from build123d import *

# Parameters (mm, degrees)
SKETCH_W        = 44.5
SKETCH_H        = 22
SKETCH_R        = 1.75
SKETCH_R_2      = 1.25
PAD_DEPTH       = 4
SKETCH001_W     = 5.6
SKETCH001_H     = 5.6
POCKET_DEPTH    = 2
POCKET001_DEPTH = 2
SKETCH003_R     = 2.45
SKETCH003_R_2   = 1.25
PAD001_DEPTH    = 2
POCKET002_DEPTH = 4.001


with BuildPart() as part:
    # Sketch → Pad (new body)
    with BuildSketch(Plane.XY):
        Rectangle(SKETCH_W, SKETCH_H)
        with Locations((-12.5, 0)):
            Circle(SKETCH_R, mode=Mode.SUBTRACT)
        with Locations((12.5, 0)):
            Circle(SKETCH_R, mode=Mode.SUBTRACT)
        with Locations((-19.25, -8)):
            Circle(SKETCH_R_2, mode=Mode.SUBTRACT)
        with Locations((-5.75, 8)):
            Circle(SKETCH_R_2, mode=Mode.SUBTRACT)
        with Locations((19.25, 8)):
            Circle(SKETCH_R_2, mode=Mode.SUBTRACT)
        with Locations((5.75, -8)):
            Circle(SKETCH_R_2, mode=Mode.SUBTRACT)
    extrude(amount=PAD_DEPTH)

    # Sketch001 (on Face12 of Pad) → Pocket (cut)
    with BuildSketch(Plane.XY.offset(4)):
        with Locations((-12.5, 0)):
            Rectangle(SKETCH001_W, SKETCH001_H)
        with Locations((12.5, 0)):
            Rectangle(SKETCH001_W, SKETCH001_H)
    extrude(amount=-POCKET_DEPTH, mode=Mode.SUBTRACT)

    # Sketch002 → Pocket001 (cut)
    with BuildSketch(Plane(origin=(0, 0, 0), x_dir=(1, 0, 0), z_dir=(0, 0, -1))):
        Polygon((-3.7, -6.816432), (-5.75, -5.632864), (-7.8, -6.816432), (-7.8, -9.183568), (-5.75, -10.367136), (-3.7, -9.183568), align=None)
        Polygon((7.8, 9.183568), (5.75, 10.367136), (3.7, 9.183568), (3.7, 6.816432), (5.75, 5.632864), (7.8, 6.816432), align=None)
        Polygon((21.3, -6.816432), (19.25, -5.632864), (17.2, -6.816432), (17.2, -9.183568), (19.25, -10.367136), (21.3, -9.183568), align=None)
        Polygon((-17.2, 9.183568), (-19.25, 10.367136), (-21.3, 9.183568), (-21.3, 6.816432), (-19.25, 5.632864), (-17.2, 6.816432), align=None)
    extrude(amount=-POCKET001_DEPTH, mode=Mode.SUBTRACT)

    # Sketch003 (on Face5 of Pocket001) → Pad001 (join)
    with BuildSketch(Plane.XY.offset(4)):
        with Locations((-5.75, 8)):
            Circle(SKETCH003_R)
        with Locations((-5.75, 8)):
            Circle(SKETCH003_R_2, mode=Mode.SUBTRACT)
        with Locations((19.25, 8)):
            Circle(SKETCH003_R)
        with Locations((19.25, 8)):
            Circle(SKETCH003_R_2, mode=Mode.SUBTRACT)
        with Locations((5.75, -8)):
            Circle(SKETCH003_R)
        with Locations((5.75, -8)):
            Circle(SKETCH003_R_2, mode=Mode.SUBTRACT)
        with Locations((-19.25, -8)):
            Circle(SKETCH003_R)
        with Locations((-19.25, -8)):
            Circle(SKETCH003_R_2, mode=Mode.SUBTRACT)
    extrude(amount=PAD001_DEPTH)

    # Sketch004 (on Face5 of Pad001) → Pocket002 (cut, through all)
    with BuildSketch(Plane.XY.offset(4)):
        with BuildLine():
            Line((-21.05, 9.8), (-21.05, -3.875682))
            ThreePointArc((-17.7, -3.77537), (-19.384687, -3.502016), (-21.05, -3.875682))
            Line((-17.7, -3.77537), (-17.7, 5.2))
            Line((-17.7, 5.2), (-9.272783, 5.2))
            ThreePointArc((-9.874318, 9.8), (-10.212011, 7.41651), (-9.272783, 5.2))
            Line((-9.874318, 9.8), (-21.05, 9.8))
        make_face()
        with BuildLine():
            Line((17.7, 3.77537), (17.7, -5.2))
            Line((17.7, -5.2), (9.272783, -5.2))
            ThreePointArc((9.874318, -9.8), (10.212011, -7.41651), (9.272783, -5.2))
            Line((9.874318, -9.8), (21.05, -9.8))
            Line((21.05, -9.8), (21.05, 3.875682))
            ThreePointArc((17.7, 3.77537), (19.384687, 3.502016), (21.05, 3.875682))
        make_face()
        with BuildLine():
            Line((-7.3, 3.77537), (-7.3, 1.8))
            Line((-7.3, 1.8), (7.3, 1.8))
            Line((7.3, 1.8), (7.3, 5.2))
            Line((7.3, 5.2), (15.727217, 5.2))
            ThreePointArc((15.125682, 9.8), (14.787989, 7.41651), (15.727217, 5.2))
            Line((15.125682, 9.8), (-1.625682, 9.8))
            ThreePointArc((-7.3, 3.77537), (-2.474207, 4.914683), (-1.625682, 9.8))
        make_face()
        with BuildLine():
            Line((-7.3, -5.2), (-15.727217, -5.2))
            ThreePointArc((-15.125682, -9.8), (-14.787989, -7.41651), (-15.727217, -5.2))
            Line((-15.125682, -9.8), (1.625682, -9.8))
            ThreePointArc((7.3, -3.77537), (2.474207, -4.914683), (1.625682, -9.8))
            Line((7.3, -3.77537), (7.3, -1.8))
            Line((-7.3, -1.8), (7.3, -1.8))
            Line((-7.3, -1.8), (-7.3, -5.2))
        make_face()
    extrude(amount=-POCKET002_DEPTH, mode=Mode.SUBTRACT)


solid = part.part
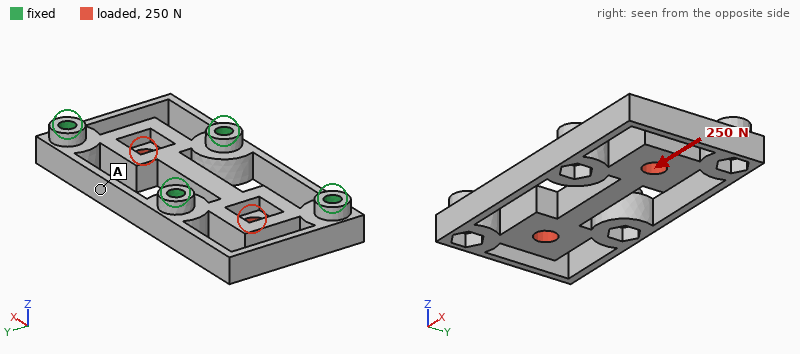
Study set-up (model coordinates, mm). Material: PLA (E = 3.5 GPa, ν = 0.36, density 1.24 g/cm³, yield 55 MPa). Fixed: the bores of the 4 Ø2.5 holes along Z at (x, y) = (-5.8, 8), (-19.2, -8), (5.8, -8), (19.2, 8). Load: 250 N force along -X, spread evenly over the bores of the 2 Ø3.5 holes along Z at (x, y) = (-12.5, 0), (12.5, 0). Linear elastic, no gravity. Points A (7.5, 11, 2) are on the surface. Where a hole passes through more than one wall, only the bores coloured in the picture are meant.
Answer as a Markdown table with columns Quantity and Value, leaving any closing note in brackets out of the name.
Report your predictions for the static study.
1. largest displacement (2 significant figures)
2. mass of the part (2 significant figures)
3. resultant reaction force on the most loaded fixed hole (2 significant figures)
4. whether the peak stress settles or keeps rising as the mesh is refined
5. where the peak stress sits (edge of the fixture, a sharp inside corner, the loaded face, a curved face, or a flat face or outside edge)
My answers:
| Quantity | Value |
|---|---|
| largest displacement | 56 µm |
| mass of the part | 2.6 g |
| resultant reaction force on the most loaded fixed hole | 64 N |
| whether the peak stress settles or keeps rising as the mesh is refined | keeps rising |
| where the peak stress sits | edge of the fixture |
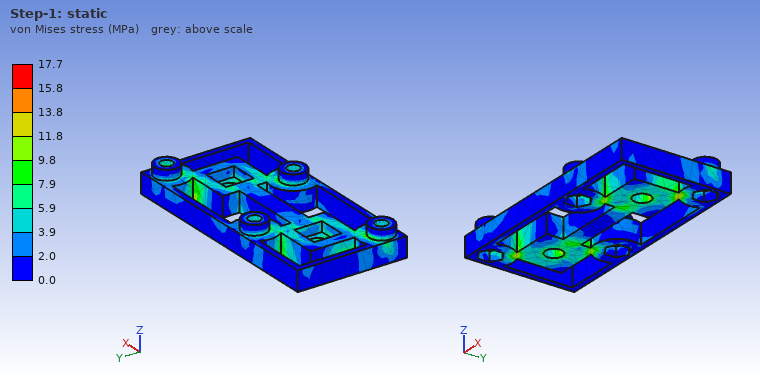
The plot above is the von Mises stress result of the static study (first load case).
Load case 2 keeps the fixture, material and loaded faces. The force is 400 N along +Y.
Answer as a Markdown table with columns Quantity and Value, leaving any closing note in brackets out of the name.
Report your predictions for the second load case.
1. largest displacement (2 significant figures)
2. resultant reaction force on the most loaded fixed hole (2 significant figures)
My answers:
| Quantity | Value |
|---|---|
| largest displacement | 82 µm |
| resultant reaction force on the most loaded fixed hole | 100 N |
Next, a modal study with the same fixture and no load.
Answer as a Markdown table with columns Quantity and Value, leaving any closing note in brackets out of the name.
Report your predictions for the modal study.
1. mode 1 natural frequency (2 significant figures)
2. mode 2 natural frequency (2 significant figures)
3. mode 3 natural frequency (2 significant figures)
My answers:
| Quantity | Value |
|---|---|
| mode 1 natural frequency | 4400 Hz |
| mode 2 natural frequency | 4400 Hz |
| mode 3 natural frequency | 6300 Hz |
